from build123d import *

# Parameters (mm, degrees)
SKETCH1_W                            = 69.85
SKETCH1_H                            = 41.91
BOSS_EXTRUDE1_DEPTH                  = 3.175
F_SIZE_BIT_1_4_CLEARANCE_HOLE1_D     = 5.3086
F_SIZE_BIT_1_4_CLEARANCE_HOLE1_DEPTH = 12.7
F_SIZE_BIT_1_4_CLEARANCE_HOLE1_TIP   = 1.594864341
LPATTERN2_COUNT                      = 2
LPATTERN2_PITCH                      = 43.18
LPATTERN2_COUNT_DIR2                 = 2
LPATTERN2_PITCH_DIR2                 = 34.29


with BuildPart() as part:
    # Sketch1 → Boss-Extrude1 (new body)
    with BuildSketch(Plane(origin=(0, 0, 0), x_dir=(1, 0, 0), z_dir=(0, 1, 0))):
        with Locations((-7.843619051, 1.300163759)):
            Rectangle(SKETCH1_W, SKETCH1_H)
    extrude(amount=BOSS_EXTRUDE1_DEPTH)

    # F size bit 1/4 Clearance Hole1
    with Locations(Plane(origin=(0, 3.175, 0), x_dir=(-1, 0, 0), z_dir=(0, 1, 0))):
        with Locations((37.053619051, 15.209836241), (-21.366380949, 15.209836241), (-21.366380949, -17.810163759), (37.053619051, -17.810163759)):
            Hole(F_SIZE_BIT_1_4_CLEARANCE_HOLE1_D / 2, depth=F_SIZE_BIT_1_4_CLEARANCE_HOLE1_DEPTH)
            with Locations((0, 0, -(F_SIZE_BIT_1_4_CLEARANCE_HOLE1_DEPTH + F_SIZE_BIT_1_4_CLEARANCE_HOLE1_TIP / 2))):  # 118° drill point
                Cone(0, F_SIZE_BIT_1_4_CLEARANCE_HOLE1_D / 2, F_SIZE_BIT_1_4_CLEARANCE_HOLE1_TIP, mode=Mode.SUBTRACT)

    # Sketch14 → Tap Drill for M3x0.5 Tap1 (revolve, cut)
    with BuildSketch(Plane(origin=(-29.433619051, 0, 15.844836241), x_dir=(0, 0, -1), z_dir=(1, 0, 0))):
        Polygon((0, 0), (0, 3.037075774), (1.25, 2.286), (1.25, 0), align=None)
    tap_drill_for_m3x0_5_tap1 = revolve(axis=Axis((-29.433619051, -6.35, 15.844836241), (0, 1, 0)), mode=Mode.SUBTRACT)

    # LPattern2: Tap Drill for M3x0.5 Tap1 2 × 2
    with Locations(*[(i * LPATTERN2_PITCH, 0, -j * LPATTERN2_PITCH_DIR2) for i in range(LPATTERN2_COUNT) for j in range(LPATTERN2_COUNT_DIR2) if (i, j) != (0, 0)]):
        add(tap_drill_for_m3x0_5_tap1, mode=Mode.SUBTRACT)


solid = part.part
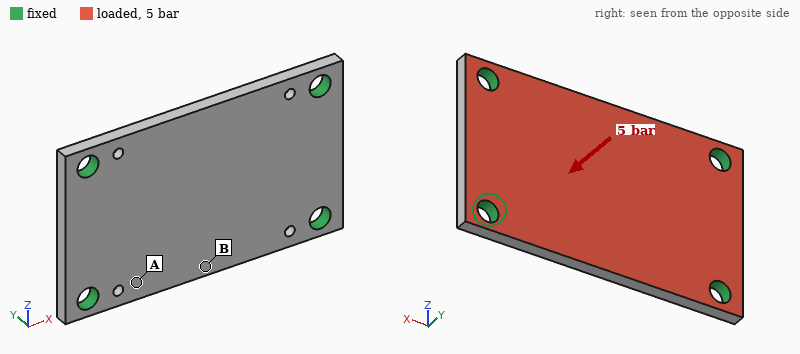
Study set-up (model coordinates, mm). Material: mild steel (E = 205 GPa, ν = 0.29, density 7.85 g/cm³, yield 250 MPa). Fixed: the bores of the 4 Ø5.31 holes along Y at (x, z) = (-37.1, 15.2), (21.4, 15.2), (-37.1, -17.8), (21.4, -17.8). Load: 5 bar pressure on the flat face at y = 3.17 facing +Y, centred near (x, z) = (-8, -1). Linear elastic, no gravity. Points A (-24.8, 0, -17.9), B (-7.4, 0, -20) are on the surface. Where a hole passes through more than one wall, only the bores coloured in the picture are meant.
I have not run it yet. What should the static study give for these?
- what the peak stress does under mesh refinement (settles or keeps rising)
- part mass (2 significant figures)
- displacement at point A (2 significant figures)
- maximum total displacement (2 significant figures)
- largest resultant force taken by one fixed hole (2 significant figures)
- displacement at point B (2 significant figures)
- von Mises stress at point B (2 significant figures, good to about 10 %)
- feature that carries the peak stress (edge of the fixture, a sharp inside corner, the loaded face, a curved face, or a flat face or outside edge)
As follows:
keeps rising
70 g
12 µm
30 µm
360 N
28 µm
46 MPa
edge of the fixture
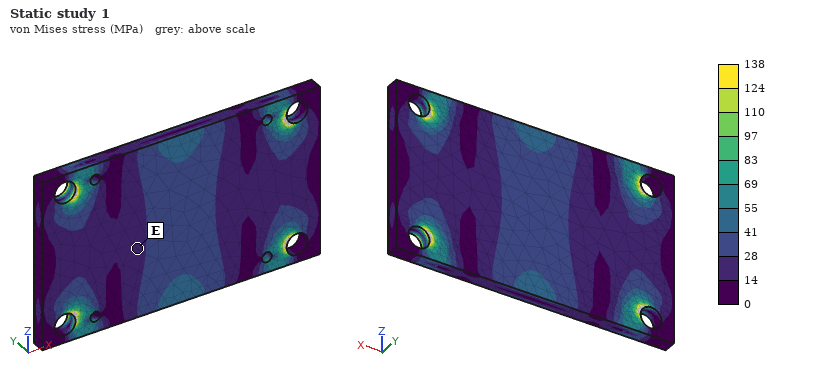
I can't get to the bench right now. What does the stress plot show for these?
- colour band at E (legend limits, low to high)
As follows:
14 to 28 MPa
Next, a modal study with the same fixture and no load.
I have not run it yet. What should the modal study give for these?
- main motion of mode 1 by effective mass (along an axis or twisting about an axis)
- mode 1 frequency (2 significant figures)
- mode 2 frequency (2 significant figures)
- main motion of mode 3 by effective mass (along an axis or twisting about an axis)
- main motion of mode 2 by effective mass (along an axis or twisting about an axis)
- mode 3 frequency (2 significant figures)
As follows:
along Y
4700 Hz
7100 Hz
twisting about Z
twisting about X
12 kHz
